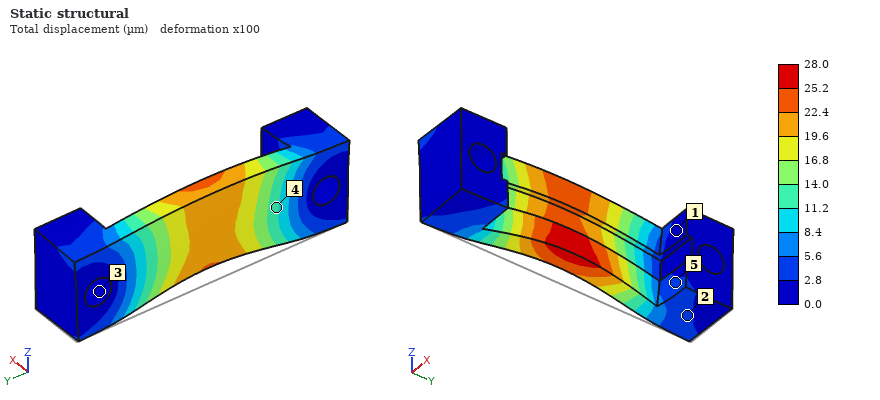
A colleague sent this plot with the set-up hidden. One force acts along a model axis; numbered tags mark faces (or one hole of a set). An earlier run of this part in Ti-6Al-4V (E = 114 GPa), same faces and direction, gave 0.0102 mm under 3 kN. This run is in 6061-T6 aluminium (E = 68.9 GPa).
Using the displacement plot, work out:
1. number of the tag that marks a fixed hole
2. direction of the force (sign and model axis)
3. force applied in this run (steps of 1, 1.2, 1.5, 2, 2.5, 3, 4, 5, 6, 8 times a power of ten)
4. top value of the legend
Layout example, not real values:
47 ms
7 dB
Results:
3
+Z
5 kN
28.0 µm
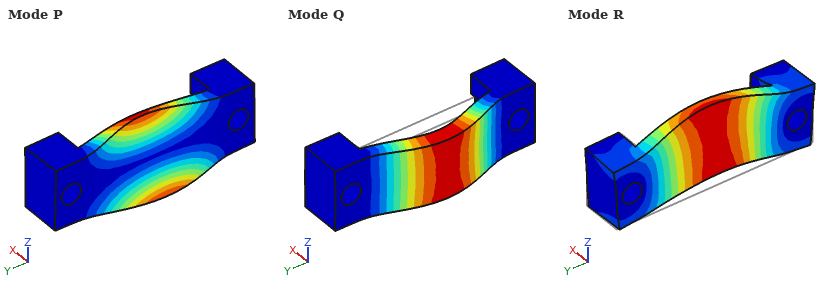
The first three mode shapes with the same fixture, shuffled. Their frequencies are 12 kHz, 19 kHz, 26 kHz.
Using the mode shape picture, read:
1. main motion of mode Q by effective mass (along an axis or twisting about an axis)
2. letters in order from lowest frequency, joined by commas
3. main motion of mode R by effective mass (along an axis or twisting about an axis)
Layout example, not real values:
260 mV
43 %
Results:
along X
Q, P, R
along Z
